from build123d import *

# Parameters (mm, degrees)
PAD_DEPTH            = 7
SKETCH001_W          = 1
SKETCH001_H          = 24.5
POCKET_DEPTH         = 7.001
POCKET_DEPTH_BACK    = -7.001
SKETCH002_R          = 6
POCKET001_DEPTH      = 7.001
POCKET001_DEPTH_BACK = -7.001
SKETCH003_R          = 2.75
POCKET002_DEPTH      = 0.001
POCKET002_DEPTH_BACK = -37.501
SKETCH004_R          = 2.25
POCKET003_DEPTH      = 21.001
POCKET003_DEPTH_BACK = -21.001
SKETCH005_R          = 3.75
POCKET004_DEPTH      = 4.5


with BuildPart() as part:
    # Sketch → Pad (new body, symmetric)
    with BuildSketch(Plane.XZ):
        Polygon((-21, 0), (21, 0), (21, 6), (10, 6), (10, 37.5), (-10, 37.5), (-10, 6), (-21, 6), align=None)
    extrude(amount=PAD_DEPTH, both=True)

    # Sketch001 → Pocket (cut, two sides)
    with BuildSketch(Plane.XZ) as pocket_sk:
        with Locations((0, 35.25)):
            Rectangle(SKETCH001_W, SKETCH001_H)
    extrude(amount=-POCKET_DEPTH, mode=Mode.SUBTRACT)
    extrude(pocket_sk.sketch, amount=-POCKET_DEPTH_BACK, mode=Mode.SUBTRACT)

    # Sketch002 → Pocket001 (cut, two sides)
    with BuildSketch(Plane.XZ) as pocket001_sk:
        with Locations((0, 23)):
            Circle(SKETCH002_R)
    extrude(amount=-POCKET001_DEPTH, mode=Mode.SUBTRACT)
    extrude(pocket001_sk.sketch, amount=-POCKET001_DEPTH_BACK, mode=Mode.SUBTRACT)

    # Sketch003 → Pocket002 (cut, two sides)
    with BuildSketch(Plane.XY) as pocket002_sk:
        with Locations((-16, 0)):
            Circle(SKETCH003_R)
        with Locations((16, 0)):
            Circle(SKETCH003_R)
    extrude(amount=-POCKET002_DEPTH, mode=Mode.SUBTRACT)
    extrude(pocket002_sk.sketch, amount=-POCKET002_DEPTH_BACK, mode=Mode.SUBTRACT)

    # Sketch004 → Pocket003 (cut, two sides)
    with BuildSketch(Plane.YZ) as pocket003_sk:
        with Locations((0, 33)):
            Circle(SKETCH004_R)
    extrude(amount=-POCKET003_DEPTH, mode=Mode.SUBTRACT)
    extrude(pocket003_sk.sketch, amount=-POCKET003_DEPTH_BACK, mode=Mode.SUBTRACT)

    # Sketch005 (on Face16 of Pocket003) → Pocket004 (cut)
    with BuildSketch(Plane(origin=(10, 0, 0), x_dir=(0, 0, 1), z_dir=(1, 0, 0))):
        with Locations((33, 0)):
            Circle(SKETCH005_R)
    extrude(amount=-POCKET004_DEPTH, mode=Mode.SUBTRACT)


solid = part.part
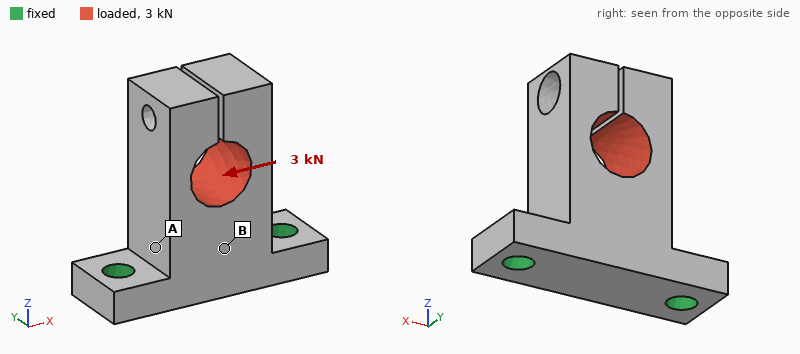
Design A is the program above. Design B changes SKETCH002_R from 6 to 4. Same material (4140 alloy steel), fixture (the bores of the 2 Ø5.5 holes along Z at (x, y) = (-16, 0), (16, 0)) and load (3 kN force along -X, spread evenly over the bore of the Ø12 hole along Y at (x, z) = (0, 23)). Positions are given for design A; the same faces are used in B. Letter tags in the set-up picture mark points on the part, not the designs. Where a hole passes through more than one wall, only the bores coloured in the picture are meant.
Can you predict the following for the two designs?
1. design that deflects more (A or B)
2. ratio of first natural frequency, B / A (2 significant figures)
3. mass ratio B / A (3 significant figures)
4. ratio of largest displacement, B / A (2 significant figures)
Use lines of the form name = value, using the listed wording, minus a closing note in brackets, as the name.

design that deflects more = A
ratio of first natural frequency, B / A = 0.96
mass ratio B / A = 1.09
ratio of largest displacement, B / A = 0.53
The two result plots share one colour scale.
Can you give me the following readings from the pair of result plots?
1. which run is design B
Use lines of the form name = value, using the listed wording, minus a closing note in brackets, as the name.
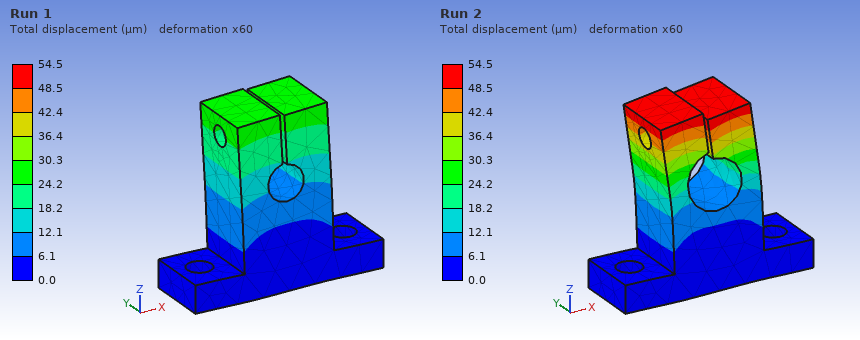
which run is design B = Run 1
